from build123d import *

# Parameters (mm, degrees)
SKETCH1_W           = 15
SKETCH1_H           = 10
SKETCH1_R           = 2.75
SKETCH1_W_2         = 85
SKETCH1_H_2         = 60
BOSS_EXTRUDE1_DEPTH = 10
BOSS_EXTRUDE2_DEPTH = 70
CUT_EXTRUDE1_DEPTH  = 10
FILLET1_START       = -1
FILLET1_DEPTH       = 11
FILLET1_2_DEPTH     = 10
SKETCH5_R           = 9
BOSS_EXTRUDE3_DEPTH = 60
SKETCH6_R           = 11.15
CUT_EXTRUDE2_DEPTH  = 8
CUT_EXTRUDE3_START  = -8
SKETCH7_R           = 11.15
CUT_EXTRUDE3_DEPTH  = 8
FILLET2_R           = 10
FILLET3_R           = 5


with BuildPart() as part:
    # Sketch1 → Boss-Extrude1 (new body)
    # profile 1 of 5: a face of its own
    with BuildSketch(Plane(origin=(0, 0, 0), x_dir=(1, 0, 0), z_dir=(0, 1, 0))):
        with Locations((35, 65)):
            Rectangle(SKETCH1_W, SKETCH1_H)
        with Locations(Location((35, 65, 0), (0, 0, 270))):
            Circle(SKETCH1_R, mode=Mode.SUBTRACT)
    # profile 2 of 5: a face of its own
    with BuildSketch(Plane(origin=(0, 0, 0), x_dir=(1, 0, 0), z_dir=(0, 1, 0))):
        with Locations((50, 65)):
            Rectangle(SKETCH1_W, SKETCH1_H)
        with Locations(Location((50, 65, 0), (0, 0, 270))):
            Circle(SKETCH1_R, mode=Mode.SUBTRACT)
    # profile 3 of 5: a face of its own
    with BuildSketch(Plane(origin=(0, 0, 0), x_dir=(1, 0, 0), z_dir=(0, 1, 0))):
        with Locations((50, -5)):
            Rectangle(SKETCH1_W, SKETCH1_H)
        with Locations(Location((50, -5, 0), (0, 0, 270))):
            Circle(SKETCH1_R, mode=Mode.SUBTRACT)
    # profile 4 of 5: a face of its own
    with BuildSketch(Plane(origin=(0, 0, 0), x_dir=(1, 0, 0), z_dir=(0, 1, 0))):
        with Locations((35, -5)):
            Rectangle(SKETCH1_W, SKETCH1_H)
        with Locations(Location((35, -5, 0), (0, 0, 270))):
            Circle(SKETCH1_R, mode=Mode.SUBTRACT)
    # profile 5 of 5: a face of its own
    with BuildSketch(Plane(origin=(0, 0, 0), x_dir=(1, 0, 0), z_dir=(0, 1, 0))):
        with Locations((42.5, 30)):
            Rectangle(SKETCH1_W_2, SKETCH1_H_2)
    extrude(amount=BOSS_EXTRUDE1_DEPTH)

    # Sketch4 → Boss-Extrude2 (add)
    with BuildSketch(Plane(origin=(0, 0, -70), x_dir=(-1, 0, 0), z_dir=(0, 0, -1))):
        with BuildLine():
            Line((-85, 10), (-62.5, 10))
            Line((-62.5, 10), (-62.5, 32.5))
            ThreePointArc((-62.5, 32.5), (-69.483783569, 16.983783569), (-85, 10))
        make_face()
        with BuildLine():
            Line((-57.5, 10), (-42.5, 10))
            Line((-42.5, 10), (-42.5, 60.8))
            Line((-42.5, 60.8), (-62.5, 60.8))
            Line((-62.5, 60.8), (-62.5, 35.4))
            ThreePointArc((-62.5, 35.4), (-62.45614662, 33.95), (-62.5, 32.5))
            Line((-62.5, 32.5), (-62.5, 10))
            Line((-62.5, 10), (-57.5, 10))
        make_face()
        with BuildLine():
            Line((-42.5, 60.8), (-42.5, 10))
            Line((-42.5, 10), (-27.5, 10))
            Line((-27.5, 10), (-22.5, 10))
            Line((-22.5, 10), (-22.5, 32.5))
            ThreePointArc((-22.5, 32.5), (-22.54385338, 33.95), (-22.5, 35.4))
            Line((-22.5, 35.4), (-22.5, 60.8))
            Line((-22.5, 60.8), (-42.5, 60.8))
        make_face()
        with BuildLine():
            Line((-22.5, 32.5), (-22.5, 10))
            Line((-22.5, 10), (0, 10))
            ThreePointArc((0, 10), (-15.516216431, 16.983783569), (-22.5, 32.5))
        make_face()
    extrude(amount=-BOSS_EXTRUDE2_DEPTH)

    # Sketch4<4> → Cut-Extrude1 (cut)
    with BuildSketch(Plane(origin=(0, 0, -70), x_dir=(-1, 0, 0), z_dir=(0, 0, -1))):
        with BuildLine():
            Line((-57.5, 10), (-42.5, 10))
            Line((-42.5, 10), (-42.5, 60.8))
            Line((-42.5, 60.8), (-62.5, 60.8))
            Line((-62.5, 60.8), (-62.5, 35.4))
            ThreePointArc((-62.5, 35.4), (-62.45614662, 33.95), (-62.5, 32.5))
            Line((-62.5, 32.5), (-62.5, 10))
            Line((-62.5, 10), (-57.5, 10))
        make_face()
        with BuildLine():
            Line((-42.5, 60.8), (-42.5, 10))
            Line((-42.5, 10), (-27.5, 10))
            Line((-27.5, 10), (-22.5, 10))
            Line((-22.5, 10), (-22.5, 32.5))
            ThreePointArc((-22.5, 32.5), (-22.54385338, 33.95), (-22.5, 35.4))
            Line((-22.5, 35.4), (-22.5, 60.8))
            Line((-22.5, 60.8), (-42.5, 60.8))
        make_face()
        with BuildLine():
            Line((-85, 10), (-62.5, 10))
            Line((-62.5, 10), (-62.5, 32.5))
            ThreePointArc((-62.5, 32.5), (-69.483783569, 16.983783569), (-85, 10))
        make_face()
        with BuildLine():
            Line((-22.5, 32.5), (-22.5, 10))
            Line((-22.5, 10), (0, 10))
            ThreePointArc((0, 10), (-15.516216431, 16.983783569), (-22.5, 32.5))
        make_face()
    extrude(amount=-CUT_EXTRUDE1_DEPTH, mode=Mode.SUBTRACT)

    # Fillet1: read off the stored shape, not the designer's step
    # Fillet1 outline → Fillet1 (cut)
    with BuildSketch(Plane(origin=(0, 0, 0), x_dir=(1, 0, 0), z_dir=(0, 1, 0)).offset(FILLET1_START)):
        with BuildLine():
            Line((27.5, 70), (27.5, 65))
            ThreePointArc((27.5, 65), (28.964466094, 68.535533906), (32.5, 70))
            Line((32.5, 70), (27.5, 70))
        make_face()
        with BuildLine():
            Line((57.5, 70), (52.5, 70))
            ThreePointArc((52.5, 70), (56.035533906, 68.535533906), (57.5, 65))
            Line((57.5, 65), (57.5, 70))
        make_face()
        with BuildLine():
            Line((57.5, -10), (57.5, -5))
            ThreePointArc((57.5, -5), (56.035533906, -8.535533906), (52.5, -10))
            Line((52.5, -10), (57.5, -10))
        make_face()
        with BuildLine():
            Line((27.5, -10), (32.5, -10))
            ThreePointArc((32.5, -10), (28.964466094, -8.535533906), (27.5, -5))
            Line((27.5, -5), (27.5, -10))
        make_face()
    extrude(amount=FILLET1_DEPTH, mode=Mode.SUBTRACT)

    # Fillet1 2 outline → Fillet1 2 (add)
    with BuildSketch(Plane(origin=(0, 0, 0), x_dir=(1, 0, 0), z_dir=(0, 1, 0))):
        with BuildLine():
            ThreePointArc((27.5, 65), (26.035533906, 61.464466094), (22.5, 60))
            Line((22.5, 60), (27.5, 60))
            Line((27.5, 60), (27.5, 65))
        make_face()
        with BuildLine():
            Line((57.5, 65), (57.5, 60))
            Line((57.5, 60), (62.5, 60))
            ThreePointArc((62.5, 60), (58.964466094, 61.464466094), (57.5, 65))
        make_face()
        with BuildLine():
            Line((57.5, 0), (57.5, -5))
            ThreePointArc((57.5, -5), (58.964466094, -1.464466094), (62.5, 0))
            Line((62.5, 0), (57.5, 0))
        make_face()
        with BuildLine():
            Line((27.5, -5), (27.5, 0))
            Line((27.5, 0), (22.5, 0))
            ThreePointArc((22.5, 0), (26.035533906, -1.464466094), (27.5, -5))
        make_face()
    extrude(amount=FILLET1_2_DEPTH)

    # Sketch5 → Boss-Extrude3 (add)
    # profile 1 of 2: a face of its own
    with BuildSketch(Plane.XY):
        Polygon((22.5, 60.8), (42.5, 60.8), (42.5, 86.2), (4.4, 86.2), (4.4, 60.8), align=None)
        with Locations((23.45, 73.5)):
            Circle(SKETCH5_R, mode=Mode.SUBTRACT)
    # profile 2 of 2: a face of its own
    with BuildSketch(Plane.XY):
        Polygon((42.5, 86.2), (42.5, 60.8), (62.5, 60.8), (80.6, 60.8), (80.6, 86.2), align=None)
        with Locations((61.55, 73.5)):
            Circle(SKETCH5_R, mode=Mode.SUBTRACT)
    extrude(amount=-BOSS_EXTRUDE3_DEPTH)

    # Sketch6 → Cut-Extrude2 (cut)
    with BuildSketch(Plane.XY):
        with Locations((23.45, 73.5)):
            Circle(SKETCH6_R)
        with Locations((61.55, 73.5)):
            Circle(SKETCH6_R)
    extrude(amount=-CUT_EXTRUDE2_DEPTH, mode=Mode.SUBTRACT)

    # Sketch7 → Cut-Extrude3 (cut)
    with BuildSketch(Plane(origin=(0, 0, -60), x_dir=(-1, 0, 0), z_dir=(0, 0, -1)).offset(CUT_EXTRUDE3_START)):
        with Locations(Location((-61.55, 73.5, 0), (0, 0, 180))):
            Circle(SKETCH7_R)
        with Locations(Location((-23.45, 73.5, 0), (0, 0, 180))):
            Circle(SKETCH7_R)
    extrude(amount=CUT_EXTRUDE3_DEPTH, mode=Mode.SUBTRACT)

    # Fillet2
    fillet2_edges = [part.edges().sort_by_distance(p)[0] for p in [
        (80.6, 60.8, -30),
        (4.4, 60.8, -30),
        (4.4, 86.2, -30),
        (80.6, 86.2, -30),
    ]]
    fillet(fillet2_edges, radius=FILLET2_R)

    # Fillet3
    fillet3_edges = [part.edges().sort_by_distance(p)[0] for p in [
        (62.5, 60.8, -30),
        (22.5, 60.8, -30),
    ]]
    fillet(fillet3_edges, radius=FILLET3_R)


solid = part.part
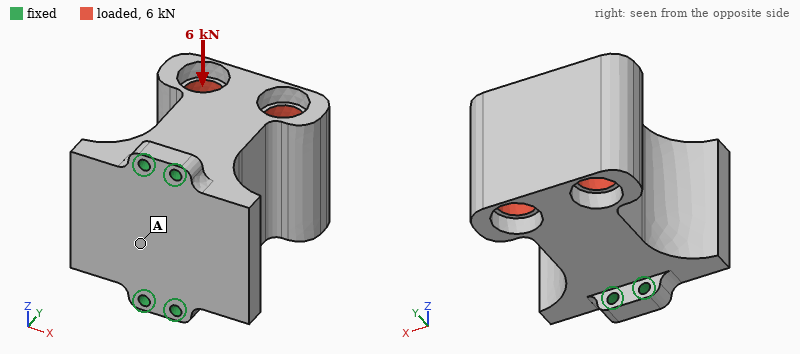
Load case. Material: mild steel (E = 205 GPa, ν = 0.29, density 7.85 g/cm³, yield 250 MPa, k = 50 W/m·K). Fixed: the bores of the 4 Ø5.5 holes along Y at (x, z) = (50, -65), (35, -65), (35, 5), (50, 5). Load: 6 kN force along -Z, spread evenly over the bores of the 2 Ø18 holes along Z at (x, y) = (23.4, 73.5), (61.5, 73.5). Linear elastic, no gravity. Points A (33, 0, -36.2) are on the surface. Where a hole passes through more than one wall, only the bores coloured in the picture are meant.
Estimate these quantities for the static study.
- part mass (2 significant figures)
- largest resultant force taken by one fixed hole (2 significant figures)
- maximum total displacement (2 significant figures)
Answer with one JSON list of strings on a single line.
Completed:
["2.1 kg", "3.6 kN", "16 µm"]
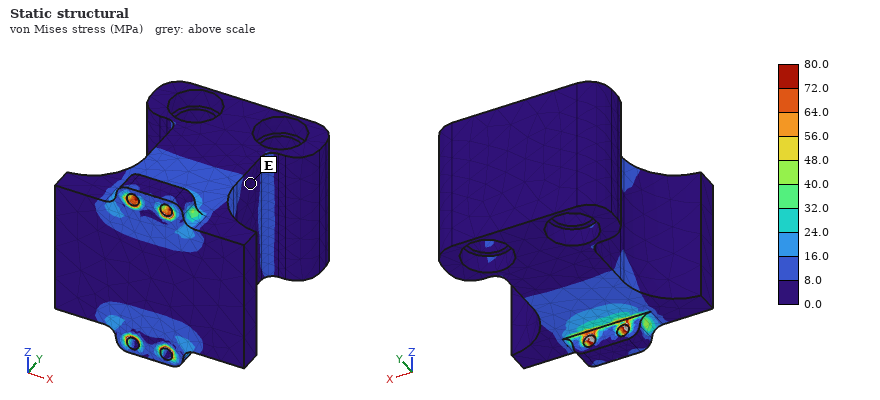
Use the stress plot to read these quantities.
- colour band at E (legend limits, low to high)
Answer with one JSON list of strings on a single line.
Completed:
["0.0 to 8.0 MPa"]
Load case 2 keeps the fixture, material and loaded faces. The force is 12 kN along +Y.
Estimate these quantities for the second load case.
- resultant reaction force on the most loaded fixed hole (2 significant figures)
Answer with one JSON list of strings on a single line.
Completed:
["3.2 kN"]
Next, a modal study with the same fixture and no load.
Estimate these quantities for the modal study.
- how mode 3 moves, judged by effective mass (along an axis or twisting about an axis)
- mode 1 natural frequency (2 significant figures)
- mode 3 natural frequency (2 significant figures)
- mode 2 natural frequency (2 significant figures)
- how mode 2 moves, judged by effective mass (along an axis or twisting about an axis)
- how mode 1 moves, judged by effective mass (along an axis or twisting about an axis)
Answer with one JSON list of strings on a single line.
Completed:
["along Y", "1400 Hz", "6100 Hz", "3800 Hz", "along Z", "along X"]
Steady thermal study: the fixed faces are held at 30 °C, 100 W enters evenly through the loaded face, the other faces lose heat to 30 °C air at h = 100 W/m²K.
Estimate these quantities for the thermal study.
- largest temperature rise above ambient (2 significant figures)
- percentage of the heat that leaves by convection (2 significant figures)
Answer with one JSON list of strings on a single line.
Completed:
["39 K", "71 %"]
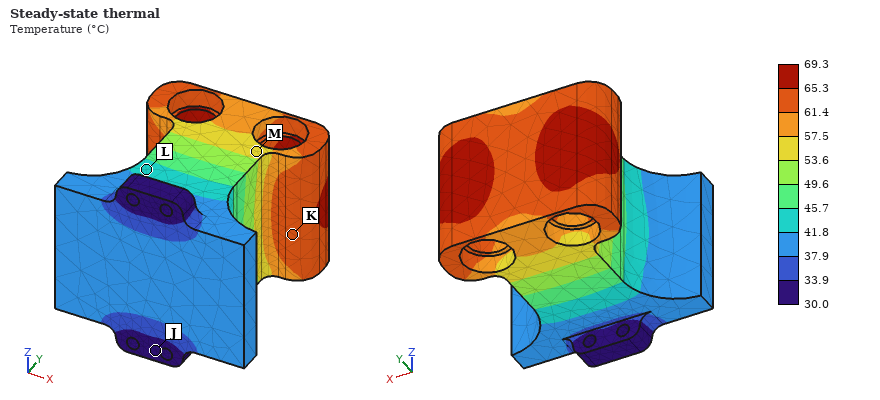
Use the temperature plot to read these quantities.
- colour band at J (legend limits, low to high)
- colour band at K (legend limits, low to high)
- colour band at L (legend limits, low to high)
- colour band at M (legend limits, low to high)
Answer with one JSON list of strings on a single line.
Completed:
["30.0 to 33.9 °C", "61.4 to 65.3 °C", "41.8 to 45.7 °C", "53.6 to 57.5 °C"]
